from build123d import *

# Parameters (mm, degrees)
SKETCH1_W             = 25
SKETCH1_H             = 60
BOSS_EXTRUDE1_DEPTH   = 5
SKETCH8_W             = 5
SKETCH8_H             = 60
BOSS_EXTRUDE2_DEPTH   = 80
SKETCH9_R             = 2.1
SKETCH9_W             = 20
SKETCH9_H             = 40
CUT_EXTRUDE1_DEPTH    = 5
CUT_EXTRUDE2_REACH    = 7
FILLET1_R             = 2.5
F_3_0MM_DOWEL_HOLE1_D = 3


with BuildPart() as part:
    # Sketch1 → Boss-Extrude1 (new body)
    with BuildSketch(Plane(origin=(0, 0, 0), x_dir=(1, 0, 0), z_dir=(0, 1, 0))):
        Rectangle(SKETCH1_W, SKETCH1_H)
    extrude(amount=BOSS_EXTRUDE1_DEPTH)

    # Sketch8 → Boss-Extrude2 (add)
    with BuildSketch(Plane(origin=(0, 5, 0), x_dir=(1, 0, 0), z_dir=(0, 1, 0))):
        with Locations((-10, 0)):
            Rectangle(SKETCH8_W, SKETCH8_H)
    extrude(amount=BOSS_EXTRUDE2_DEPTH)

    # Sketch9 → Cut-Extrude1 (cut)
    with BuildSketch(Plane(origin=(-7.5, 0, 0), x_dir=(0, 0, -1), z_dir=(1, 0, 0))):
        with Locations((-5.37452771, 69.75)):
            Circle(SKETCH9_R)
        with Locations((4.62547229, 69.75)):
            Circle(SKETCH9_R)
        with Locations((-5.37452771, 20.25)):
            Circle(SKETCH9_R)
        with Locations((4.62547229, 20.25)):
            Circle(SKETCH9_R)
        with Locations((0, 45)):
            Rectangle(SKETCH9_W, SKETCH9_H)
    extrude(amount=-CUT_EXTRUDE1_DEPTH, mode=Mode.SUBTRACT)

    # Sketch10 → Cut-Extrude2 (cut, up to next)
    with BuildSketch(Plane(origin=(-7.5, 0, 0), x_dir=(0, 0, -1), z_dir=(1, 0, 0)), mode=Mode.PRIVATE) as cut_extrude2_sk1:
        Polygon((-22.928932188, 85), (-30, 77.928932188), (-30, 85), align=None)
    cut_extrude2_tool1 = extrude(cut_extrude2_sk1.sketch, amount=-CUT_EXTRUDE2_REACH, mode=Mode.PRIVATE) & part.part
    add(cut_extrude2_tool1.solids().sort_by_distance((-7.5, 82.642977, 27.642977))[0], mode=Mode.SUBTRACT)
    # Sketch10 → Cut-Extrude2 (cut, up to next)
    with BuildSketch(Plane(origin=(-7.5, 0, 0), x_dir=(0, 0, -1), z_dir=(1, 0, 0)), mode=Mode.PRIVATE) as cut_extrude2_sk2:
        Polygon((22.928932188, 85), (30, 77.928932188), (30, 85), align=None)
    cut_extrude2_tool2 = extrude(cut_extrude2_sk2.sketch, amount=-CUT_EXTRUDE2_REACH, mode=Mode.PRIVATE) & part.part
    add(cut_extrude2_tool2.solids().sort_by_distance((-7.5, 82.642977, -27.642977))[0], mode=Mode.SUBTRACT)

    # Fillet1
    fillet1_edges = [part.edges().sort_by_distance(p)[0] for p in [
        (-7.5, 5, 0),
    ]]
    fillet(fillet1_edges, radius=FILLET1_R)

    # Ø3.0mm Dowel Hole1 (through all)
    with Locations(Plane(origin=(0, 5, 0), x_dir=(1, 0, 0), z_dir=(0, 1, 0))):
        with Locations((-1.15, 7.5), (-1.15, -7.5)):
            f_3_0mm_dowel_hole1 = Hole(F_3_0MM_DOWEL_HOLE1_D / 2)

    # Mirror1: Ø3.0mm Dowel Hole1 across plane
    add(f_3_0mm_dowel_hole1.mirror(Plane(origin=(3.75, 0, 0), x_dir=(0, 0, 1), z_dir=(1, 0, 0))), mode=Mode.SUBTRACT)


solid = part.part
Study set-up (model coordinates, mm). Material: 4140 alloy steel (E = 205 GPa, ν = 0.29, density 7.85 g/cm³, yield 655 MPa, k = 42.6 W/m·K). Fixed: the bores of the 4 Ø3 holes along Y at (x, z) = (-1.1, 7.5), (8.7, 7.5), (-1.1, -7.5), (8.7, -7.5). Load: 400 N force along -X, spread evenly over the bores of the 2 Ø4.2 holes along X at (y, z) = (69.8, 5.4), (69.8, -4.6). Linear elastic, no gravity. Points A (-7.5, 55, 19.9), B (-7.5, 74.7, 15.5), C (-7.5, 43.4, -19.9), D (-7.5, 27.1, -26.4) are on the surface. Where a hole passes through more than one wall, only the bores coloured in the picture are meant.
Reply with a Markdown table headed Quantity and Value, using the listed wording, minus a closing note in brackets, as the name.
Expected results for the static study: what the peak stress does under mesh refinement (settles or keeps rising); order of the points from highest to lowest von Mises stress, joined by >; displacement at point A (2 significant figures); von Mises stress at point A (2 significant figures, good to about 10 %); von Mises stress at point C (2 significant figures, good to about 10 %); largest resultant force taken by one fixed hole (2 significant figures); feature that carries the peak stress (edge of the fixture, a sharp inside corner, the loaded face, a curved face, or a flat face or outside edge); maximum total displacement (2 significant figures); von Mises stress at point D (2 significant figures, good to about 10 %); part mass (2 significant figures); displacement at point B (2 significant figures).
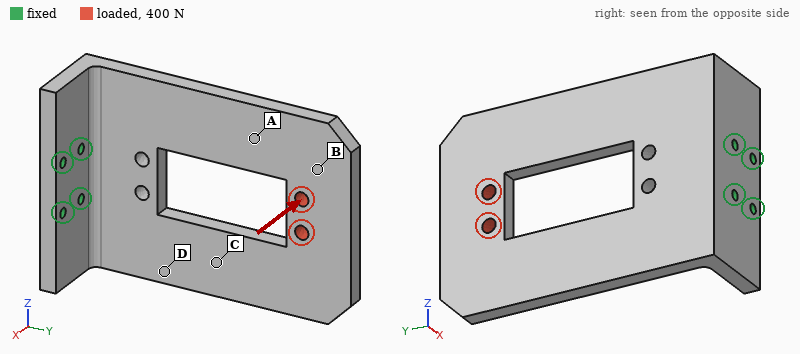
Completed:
| Quantity | Value |
|---|---|
| what the peak stress does under mesh refinement | keeps rising |
| order of the points from highest to lowest von Mises stress, joined by > | D > C > A > B |
| displacement at point A | 0.34 mm |
| von Mises stress at point A | 37 MPa |
| von Mises stress at point C | 65 MPa |
| largest resultant force taken by one fixed hole | 650 N |
| feature that carries the peak stress | edge of the fixture |
| maximum total displacement | 0.66 mm |
| von Mises stress at point D | 94 MPa |
| part mass | 210 g |
| displacement at point B | 0.55 mm |
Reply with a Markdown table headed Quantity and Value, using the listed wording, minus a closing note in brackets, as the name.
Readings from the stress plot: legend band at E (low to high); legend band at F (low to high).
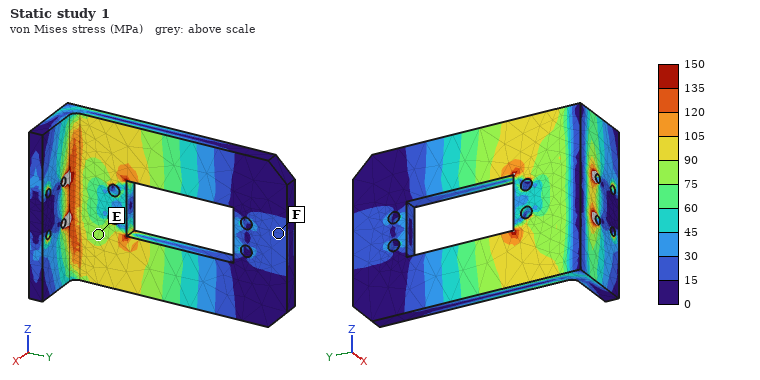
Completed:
| Quantity | Value |
|---|---|
| legend band at E | 75 to 90 MPa |
| legend band at F | 15 to 30 MPa |
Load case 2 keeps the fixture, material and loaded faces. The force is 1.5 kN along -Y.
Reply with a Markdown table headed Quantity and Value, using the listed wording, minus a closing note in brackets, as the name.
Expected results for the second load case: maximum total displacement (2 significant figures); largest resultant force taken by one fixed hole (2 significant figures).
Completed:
| Quantity | Value |
|---|---|
| maximum total displacement | 59 µm |
| largest resultant force taken by one fixed hole | 1.0 kN |
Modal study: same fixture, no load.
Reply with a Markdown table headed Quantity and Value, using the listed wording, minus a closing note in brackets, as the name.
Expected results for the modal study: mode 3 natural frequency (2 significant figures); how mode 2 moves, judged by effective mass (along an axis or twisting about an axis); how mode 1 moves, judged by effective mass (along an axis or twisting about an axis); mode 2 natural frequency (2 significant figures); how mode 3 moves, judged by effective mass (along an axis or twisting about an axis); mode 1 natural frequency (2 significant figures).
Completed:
| Quantity | Value |
|---|---|
| mode 3 natural frequency | 1700 Hz |
| how mode 2 moves, judged by effective mass | along Z |
| how mode 1 moves, judged by effective mass | along X |
| mode 2 natural frequency | 1400 Hz |
| how mode 3 moves, judged by effective mass | along Z |
| mode 1 natural frequency | 530 Hz |
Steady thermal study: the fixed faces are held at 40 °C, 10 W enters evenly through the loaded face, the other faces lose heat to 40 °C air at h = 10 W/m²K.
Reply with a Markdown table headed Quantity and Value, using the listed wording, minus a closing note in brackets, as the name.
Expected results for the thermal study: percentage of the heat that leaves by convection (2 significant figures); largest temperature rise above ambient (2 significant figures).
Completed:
| Quantity | Value |
|---|---|
| percentage of the heat that leaves by convection | 37 % |
| largest temperature rise above ambient | 78 K |
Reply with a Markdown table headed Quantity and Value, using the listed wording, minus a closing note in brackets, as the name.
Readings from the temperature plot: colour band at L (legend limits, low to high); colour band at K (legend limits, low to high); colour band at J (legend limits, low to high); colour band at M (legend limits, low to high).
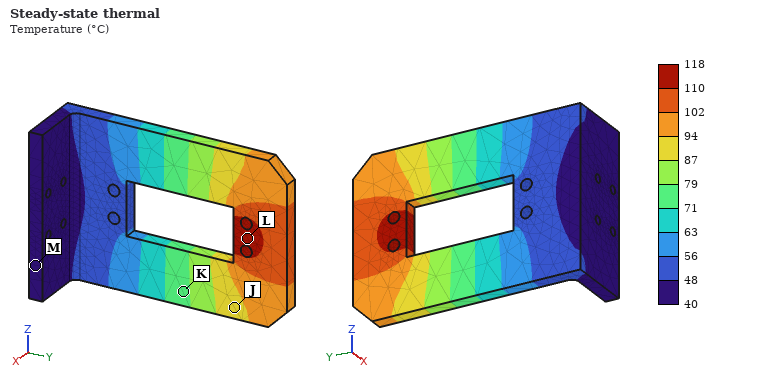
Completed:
| Quantity | Value |
|---|---|
| colour band at L | 110 to 118 °C |
| colour band at K | 71 to 79 °C |
| colour band at J | 87 to 94 °C |
| colour band at M | 40 to 48 °C |
